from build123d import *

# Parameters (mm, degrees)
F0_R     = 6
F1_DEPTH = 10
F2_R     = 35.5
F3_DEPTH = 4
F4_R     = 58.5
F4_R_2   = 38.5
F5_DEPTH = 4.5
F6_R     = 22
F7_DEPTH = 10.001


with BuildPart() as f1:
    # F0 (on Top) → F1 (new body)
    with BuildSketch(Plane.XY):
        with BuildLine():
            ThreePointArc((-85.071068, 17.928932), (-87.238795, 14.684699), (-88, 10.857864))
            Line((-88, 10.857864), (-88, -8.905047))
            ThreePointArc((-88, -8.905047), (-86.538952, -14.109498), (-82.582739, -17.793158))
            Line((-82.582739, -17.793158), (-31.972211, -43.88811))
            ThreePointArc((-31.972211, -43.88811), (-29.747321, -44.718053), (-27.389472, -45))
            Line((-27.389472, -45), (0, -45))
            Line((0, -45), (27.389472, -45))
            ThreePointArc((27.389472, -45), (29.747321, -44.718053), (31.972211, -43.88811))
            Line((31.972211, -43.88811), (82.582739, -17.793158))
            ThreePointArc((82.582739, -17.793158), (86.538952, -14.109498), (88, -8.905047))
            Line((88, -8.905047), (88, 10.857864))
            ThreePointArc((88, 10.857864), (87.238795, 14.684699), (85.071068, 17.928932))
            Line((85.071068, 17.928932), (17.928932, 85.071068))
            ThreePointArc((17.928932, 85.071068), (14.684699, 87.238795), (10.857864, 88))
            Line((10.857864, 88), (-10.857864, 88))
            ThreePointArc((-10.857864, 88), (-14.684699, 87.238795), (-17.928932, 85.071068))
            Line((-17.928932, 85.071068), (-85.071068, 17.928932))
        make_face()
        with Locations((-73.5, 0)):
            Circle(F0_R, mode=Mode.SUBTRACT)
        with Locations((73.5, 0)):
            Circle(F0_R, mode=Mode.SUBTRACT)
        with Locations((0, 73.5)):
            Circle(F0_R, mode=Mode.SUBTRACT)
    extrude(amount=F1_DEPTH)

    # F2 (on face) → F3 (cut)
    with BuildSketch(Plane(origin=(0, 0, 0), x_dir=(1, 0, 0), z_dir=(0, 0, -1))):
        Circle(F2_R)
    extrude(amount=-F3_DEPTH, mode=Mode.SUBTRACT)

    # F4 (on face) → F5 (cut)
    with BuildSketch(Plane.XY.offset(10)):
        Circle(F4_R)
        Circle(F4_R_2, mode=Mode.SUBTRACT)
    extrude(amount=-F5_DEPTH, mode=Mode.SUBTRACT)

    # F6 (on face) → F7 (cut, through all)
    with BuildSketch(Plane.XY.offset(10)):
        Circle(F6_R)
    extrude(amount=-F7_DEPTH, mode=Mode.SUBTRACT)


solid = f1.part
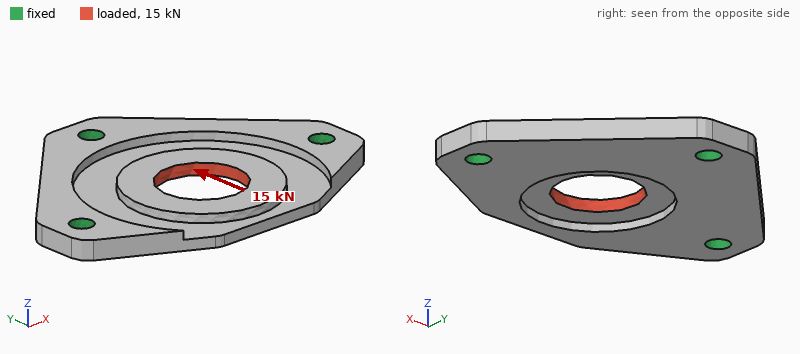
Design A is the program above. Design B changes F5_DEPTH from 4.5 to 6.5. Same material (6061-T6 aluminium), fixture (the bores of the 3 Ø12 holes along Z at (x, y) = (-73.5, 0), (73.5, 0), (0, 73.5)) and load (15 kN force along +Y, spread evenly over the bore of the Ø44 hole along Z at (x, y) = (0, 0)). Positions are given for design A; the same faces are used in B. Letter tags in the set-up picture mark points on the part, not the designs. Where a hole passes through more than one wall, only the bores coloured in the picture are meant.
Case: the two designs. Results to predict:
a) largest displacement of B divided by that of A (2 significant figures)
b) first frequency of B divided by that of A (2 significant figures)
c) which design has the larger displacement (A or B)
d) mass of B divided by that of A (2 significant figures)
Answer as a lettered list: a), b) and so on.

a) 2.0
b) 0.91
c) B
d) 0.90
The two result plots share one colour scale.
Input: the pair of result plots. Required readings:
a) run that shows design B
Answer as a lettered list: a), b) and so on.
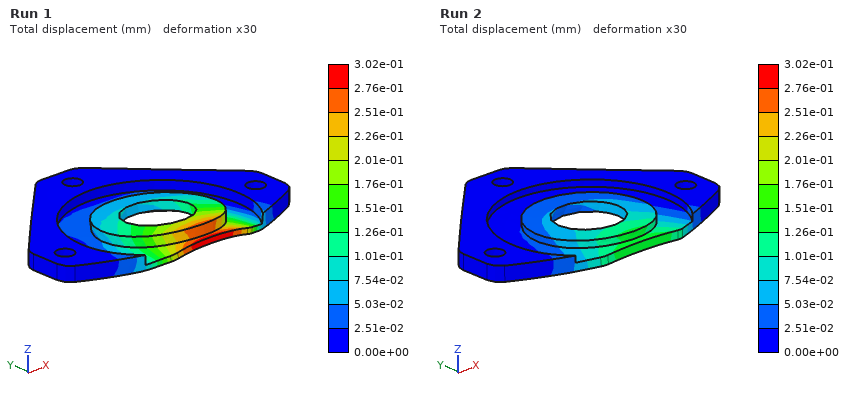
a) Run 1
